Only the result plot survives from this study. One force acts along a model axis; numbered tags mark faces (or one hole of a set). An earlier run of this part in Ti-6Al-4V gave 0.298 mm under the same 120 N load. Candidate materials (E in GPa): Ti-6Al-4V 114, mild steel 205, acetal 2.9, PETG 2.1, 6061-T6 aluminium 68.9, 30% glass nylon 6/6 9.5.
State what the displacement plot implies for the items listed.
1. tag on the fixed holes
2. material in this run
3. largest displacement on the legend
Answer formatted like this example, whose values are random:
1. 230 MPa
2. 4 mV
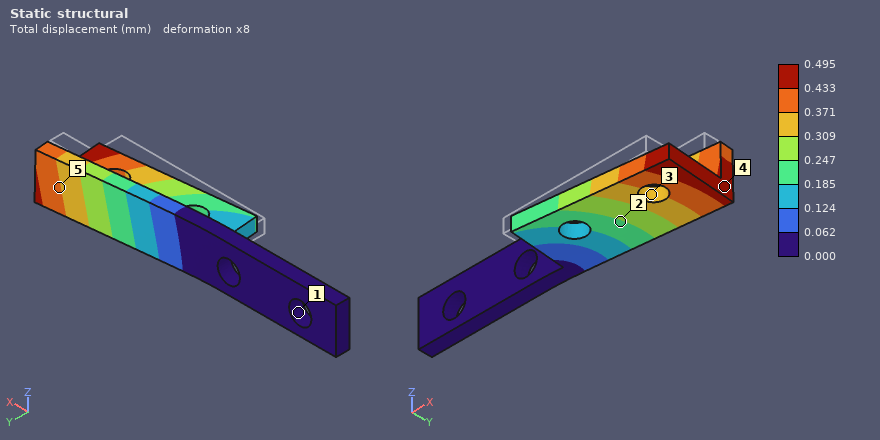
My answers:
1. 1
2. 6061-T6 aluminium
3. 0.495 mm
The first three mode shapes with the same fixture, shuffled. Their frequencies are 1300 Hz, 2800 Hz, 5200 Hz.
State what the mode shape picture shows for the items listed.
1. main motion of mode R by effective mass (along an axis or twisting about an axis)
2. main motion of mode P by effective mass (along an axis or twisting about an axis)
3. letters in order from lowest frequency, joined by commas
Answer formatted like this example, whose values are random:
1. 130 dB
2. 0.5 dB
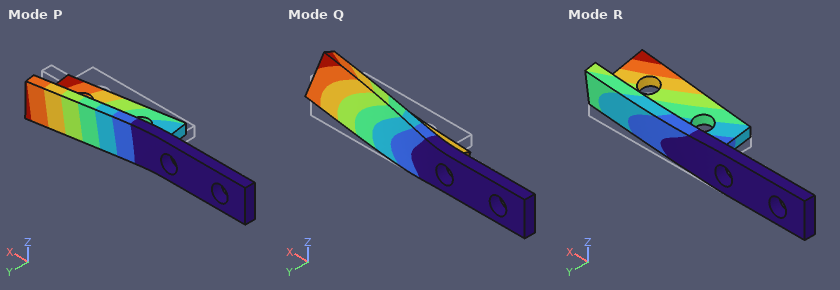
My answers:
1. along Z
2. along Y
3. P, R, Q
